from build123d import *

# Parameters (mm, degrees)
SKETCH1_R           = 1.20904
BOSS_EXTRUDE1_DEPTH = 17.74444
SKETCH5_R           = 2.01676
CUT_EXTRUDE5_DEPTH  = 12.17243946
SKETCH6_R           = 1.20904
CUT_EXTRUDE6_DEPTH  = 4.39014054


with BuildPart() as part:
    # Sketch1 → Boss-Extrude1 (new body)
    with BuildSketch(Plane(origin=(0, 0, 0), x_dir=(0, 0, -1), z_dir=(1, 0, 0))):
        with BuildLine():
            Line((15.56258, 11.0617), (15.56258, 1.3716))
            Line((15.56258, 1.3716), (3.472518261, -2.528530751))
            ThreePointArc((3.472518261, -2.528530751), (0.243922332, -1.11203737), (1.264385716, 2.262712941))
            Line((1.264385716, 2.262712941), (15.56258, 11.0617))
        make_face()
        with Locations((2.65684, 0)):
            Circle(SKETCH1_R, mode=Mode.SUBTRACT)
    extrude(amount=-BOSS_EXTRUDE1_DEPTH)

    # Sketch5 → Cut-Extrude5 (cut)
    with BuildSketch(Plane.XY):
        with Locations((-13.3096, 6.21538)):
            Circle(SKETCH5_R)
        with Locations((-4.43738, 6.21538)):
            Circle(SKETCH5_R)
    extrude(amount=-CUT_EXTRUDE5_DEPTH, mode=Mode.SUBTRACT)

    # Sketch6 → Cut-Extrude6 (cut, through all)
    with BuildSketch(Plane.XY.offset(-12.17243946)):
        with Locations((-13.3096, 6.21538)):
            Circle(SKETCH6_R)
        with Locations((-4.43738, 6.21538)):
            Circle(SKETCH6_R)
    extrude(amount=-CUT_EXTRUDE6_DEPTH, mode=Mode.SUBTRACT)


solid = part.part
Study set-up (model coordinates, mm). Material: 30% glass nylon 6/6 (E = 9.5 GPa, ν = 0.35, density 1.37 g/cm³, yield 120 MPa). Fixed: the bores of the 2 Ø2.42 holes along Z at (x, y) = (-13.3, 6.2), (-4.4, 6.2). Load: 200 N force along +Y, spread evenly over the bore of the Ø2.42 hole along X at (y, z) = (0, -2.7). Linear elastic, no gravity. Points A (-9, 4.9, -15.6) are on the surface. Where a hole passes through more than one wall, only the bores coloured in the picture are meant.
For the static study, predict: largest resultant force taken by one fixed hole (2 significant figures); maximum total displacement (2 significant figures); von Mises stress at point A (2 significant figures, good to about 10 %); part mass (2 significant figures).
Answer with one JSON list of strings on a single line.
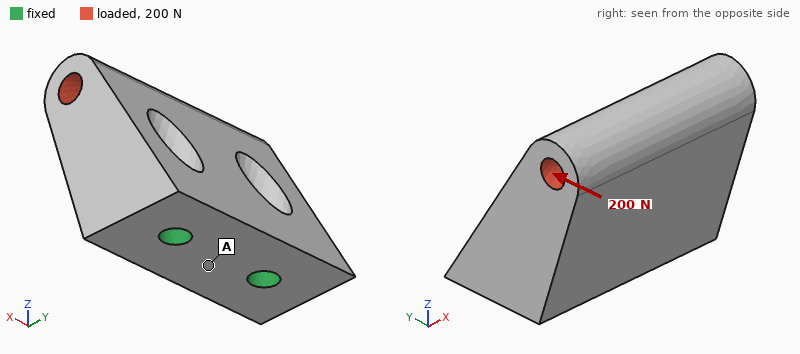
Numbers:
["100 N", "0.12 mm", "9.1 MPa", "2.4 g"]
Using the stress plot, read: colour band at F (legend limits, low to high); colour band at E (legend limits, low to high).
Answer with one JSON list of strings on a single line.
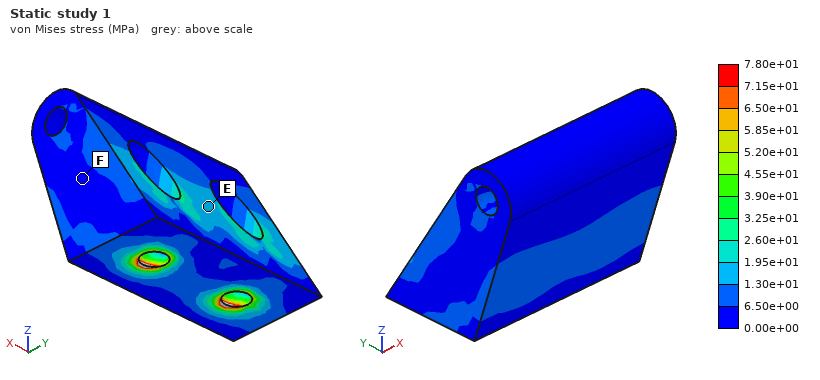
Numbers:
["0.00e+00 to 6.50e+00 MPa", "1.30e+01 to 1.95e+01 MPa"]
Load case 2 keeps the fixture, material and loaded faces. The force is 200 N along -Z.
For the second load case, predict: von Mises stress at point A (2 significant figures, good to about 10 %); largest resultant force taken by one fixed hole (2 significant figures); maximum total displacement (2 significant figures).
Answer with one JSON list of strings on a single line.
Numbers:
["5.0 MPa", "100 N", "59 µm"]
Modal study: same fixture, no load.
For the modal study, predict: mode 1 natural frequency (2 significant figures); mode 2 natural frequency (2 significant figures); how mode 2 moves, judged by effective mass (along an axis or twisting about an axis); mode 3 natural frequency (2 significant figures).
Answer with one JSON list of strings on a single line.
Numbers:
["7800 Hz", "14 kHz", "along X", "18 kHz"]
